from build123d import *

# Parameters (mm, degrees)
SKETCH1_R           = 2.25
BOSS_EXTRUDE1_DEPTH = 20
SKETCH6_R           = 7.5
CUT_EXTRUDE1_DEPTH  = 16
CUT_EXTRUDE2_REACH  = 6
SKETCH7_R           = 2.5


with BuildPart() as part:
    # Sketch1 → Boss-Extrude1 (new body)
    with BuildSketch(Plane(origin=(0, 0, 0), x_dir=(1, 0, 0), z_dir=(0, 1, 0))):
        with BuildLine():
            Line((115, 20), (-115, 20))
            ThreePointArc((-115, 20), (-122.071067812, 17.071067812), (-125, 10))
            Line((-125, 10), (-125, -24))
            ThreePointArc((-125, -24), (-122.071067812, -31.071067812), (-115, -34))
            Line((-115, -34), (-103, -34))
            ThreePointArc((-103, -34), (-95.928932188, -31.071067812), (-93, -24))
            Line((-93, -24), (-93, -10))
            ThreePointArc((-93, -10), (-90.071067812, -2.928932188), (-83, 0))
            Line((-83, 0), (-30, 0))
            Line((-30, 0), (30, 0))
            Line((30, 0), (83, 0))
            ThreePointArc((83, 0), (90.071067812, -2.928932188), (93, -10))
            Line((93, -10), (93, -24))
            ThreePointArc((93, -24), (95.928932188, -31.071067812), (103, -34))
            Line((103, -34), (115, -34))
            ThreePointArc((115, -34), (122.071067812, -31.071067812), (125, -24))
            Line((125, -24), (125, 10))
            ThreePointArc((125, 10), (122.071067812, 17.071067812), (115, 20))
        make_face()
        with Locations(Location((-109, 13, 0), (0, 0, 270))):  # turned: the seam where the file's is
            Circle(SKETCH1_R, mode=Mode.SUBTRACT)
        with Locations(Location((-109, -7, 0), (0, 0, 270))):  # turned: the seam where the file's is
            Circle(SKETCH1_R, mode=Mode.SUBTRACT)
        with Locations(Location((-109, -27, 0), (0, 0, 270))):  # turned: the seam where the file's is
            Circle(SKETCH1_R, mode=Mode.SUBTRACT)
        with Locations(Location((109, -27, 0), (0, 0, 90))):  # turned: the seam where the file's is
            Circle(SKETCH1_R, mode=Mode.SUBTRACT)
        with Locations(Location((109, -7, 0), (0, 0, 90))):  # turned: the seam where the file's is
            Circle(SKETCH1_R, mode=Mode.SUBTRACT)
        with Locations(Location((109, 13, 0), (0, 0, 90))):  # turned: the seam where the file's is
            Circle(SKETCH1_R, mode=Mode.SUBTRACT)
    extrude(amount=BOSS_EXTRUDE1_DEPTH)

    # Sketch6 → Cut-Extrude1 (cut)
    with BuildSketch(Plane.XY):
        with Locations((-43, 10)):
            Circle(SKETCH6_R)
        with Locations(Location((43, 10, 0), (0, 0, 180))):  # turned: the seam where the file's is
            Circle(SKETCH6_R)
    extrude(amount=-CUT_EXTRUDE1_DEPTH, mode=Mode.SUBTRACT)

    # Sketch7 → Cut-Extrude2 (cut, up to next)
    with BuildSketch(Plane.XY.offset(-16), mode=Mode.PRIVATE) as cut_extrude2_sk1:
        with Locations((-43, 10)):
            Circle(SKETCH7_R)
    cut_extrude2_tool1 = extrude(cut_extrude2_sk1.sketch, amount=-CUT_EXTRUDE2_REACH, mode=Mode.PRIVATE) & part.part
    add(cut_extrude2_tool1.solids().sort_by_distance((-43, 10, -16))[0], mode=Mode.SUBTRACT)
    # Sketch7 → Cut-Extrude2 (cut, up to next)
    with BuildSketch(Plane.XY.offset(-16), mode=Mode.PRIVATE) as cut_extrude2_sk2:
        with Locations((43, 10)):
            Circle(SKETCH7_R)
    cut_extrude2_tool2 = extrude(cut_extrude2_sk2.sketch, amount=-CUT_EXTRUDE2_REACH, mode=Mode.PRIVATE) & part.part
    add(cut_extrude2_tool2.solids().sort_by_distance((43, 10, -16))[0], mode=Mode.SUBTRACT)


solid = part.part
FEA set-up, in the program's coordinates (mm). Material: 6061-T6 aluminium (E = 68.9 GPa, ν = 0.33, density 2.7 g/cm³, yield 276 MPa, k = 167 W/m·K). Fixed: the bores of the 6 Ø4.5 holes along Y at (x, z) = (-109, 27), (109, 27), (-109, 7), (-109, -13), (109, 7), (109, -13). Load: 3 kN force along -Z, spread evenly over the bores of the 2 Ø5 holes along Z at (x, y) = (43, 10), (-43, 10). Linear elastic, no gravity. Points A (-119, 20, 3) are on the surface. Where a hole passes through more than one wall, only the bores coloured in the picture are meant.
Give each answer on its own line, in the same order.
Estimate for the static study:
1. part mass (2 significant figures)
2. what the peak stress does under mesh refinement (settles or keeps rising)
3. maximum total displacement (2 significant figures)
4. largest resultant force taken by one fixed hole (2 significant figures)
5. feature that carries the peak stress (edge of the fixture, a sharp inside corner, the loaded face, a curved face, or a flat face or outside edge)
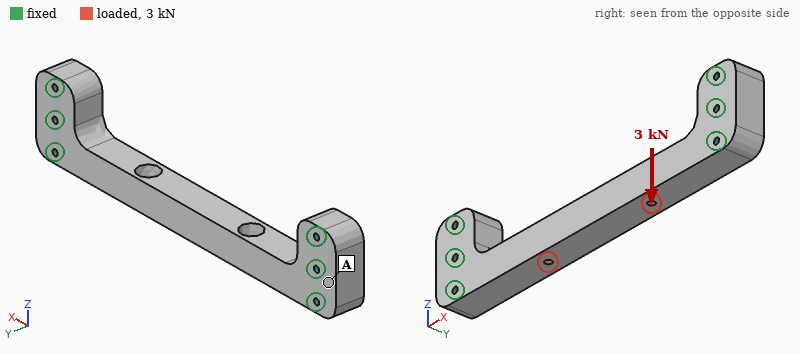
360 g
keeps rising
89 µm
2.5 kN
a sharp inside corner
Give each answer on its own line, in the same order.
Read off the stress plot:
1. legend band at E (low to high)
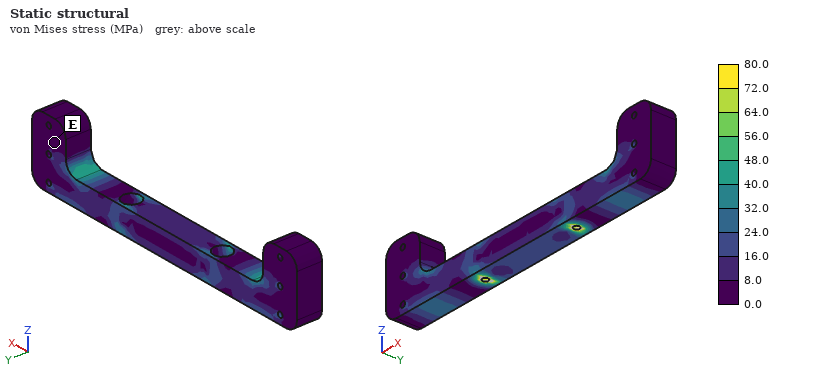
0.0 to 8.0 MPa
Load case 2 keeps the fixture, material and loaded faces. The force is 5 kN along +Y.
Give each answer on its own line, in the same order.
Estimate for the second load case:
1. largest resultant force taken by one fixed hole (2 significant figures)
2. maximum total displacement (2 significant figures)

2.0 kN
0.22 mm
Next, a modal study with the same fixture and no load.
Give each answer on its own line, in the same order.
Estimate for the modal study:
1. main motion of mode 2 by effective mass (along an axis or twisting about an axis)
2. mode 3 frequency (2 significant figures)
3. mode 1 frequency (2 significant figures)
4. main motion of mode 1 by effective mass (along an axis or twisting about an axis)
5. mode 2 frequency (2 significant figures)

along Z
5800 Hz
2200 Hz
along Y
2600 Hz
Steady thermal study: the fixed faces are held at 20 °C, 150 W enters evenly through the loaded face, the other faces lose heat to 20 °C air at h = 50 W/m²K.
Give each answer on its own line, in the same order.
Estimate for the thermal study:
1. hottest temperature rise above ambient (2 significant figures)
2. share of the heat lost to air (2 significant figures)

85 K
25 %
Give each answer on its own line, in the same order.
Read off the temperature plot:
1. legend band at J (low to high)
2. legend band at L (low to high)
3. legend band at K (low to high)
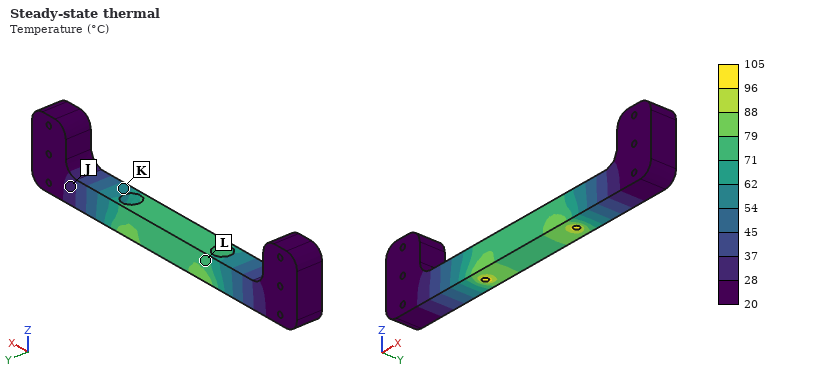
28 to 37 °C
71 to 79 °C
54 to 62 °C
